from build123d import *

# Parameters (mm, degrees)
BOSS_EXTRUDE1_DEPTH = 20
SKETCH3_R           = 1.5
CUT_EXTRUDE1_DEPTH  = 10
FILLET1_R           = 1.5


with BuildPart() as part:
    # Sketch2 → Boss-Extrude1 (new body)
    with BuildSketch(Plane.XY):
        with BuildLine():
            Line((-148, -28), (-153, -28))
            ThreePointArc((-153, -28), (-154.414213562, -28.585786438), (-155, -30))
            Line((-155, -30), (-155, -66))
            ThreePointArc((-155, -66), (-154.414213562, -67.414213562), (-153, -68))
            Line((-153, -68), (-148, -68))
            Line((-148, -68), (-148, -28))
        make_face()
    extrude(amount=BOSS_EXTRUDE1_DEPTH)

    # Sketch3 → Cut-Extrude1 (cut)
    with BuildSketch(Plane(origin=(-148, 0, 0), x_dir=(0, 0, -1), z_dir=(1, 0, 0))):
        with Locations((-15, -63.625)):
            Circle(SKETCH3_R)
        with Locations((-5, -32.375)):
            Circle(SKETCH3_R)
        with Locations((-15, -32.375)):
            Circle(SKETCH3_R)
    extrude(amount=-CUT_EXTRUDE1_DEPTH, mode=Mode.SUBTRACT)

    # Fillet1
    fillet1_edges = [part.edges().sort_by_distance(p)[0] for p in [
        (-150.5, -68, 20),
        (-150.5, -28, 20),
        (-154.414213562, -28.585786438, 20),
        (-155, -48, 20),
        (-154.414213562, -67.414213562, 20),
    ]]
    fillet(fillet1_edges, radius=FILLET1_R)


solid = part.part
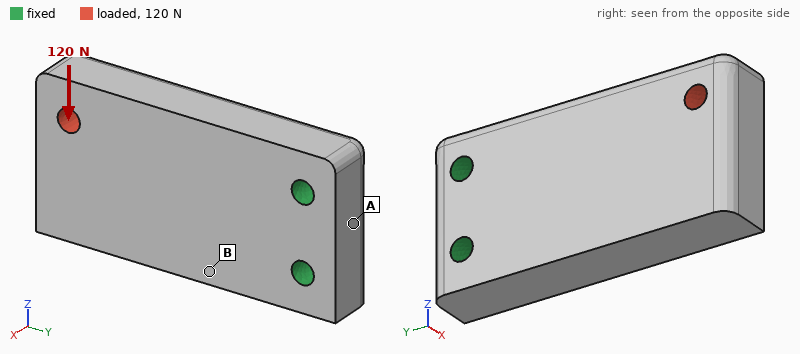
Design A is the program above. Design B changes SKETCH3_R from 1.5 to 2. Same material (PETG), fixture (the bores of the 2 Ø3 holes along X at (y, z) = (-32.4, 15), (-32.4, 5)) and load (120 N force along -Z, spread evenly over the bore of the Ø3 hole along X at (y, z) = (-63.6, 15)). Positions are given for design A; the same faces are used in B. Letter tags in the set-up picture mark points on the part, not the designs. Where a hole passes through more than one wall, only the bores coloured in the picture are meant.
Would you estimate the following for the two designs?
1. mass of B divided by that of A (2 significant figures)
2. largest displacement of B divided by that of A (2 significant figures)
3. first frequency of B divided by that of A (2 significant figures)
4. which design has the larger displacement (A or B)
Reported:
0.98
0.92
1.1
A
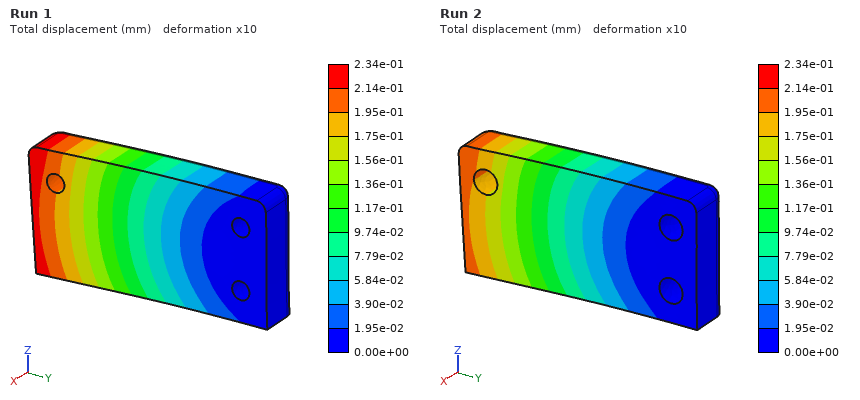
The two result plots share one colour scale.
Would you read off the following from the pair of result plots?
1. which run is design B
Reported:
Run 2
